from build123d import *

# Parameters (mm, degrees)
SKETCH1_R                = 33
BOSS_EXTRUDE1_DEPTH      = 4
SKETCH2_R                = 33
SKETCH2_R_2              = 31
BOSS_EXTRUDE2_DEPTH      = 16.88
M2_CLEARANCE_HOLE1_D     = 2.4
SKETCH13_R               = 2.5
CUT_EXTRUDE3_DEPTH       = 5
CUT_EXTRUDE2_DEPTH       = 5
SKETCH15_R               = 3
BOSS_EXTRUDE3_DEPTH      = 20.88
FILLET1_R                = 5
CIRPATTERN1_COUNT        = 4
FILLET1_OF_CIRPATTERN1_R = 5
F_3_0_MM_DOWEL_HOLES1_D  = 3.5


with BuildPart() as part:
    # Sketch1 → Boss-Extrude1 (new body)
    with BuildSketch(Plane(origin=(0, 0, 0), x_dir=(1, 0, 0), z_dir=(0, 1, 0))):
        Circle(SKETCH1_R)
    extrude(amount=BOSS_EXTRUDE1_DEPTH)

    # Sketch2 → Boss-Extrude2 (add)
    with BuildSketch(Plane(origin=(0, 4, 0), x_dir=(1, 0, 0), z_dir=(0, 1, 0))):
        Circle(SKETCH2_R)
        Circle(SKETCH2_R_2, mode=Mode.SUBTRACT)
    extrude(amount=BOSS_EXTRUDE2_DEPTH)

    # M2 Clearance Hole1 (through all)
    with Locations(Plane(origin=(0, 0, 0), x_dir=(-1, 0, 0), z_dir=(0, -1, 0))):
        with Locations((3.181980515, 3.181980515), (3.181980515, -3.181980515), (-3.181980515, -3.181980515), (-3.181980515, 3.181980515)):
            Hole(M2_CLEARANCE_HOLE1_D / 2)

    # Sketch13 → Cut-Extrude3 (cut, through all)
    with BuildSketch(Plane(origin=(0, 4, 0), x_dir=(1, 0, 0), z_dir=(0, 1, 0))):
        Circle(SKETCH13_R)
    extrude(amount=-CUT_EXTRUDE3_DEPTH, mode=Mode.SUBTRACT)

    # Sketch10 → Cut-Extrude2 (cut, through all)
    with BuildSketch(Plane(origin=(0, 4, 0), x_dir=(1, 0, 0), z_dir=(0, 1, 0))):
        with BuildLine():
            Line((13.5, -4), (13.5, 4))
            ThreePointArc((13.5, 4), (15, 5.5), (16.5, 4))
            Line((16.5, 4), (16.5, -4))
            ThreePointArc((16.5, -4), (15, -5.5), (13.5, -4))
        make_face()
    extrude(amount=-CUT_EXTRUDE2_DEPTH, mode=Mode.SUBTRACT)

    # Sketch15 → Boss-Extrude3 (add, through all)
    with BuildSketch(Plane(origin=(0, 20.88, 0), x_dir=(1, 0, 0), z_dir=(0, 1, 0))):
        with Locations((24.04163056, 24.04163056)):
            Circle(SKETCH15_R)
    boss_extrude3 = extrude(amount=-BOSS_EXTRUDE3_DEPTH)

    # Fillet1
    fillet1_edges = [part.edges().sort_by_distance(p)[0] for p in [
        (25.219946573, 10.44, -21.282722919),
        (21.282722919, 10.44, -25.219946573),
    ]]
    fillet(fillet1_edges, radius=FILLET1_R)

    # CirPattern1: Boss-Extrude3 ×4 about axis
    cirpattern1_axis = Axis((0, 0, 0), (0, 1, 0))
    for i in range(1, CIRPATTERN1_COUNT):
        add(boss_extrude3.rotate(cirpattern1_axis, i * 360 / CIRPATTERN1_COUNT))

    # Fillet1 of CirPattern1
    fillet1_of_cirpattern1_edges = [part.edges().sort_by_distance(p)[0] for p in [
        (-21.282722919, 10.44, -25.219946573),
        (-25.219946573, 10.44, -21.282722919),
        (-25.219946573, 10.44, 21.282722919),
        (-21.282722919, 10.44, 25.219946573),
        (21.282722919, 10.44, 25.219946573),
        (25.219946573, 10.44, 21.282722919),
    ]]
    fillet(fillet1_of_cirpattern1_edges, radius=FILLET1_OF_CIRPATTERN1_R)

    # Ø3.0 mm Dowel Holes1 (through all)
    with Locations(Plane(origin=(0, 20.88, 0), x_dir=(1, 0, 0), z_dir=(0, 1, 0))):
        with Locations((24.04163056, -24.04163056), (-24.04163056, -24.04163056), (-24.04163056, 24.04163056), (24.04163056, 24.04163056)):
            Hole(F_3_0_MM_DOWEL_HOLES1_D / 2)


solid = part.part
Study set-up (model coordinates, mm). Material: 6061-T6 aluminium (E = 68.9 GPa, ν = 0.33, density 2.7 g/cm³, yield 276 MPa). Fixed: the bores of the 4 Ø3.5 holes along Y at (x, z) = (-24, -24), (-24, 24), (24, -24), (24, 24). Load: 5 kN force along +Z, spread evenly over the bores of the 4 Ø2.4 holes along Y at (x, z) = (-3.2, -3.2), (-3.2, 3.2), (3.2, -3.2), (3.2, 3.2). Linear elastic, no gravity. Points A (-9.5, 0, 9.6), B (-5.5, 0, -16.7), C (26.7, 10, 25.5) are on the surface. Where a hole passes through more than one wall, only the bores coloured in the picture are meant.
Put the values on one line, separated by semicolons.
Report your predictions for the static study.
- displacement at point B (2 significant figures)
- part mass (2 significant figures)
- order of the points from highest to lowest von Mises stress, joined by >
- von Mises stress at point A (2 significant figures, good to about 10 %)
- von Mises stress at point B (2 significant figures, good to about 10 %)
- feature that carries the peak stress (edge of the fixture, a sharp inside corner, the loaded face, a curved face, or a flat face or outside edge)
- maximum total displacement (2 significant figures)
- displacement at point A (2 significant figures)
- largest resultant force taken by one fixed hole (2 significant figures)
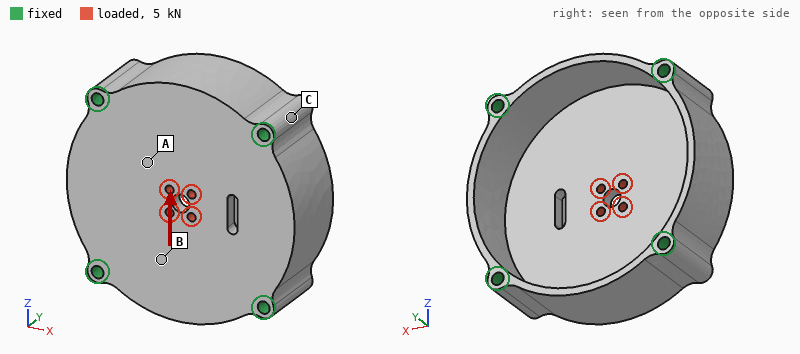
9.9 µm; 58 g; A > B > C; 25 MPa; 15 MPa; the loaded face; 18 µm; 9.2 µm; 1.4 kN
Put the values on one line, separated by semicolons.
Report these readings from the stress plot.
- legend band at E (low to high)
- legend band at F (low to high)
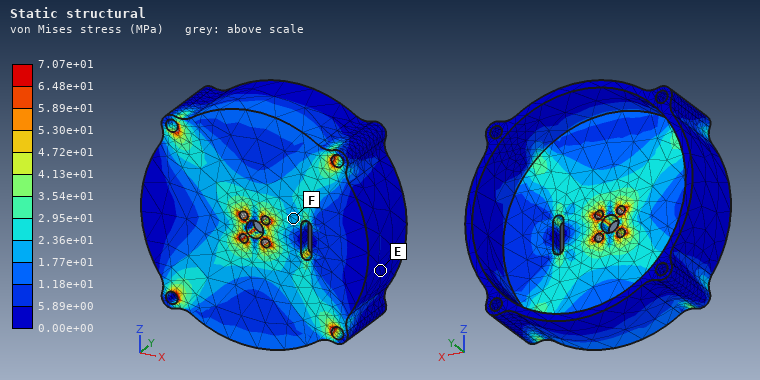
0.00e+00 to 5.89e+00 MPa; 1.77e+01 to 2.36e+01 MPa
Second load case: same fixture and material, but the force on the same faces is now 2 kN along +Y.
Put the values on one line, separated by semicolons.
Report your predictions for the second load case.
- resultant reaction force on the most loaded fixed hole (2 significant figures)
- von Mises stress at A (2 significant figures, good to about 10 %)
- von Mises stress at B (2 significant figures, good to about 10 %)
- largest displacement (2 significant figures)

510 N; 64 MPa; 50 MPa; 0.17 mm
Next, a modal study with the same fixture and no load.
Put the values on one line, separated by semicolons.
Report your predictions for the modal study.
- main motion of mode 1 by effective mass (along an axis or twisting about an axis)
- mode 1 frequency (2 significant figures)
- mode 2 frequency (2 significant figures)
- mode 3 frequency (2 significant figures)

along Y; 7000 Hz; 14 kHz; 14 kHz
